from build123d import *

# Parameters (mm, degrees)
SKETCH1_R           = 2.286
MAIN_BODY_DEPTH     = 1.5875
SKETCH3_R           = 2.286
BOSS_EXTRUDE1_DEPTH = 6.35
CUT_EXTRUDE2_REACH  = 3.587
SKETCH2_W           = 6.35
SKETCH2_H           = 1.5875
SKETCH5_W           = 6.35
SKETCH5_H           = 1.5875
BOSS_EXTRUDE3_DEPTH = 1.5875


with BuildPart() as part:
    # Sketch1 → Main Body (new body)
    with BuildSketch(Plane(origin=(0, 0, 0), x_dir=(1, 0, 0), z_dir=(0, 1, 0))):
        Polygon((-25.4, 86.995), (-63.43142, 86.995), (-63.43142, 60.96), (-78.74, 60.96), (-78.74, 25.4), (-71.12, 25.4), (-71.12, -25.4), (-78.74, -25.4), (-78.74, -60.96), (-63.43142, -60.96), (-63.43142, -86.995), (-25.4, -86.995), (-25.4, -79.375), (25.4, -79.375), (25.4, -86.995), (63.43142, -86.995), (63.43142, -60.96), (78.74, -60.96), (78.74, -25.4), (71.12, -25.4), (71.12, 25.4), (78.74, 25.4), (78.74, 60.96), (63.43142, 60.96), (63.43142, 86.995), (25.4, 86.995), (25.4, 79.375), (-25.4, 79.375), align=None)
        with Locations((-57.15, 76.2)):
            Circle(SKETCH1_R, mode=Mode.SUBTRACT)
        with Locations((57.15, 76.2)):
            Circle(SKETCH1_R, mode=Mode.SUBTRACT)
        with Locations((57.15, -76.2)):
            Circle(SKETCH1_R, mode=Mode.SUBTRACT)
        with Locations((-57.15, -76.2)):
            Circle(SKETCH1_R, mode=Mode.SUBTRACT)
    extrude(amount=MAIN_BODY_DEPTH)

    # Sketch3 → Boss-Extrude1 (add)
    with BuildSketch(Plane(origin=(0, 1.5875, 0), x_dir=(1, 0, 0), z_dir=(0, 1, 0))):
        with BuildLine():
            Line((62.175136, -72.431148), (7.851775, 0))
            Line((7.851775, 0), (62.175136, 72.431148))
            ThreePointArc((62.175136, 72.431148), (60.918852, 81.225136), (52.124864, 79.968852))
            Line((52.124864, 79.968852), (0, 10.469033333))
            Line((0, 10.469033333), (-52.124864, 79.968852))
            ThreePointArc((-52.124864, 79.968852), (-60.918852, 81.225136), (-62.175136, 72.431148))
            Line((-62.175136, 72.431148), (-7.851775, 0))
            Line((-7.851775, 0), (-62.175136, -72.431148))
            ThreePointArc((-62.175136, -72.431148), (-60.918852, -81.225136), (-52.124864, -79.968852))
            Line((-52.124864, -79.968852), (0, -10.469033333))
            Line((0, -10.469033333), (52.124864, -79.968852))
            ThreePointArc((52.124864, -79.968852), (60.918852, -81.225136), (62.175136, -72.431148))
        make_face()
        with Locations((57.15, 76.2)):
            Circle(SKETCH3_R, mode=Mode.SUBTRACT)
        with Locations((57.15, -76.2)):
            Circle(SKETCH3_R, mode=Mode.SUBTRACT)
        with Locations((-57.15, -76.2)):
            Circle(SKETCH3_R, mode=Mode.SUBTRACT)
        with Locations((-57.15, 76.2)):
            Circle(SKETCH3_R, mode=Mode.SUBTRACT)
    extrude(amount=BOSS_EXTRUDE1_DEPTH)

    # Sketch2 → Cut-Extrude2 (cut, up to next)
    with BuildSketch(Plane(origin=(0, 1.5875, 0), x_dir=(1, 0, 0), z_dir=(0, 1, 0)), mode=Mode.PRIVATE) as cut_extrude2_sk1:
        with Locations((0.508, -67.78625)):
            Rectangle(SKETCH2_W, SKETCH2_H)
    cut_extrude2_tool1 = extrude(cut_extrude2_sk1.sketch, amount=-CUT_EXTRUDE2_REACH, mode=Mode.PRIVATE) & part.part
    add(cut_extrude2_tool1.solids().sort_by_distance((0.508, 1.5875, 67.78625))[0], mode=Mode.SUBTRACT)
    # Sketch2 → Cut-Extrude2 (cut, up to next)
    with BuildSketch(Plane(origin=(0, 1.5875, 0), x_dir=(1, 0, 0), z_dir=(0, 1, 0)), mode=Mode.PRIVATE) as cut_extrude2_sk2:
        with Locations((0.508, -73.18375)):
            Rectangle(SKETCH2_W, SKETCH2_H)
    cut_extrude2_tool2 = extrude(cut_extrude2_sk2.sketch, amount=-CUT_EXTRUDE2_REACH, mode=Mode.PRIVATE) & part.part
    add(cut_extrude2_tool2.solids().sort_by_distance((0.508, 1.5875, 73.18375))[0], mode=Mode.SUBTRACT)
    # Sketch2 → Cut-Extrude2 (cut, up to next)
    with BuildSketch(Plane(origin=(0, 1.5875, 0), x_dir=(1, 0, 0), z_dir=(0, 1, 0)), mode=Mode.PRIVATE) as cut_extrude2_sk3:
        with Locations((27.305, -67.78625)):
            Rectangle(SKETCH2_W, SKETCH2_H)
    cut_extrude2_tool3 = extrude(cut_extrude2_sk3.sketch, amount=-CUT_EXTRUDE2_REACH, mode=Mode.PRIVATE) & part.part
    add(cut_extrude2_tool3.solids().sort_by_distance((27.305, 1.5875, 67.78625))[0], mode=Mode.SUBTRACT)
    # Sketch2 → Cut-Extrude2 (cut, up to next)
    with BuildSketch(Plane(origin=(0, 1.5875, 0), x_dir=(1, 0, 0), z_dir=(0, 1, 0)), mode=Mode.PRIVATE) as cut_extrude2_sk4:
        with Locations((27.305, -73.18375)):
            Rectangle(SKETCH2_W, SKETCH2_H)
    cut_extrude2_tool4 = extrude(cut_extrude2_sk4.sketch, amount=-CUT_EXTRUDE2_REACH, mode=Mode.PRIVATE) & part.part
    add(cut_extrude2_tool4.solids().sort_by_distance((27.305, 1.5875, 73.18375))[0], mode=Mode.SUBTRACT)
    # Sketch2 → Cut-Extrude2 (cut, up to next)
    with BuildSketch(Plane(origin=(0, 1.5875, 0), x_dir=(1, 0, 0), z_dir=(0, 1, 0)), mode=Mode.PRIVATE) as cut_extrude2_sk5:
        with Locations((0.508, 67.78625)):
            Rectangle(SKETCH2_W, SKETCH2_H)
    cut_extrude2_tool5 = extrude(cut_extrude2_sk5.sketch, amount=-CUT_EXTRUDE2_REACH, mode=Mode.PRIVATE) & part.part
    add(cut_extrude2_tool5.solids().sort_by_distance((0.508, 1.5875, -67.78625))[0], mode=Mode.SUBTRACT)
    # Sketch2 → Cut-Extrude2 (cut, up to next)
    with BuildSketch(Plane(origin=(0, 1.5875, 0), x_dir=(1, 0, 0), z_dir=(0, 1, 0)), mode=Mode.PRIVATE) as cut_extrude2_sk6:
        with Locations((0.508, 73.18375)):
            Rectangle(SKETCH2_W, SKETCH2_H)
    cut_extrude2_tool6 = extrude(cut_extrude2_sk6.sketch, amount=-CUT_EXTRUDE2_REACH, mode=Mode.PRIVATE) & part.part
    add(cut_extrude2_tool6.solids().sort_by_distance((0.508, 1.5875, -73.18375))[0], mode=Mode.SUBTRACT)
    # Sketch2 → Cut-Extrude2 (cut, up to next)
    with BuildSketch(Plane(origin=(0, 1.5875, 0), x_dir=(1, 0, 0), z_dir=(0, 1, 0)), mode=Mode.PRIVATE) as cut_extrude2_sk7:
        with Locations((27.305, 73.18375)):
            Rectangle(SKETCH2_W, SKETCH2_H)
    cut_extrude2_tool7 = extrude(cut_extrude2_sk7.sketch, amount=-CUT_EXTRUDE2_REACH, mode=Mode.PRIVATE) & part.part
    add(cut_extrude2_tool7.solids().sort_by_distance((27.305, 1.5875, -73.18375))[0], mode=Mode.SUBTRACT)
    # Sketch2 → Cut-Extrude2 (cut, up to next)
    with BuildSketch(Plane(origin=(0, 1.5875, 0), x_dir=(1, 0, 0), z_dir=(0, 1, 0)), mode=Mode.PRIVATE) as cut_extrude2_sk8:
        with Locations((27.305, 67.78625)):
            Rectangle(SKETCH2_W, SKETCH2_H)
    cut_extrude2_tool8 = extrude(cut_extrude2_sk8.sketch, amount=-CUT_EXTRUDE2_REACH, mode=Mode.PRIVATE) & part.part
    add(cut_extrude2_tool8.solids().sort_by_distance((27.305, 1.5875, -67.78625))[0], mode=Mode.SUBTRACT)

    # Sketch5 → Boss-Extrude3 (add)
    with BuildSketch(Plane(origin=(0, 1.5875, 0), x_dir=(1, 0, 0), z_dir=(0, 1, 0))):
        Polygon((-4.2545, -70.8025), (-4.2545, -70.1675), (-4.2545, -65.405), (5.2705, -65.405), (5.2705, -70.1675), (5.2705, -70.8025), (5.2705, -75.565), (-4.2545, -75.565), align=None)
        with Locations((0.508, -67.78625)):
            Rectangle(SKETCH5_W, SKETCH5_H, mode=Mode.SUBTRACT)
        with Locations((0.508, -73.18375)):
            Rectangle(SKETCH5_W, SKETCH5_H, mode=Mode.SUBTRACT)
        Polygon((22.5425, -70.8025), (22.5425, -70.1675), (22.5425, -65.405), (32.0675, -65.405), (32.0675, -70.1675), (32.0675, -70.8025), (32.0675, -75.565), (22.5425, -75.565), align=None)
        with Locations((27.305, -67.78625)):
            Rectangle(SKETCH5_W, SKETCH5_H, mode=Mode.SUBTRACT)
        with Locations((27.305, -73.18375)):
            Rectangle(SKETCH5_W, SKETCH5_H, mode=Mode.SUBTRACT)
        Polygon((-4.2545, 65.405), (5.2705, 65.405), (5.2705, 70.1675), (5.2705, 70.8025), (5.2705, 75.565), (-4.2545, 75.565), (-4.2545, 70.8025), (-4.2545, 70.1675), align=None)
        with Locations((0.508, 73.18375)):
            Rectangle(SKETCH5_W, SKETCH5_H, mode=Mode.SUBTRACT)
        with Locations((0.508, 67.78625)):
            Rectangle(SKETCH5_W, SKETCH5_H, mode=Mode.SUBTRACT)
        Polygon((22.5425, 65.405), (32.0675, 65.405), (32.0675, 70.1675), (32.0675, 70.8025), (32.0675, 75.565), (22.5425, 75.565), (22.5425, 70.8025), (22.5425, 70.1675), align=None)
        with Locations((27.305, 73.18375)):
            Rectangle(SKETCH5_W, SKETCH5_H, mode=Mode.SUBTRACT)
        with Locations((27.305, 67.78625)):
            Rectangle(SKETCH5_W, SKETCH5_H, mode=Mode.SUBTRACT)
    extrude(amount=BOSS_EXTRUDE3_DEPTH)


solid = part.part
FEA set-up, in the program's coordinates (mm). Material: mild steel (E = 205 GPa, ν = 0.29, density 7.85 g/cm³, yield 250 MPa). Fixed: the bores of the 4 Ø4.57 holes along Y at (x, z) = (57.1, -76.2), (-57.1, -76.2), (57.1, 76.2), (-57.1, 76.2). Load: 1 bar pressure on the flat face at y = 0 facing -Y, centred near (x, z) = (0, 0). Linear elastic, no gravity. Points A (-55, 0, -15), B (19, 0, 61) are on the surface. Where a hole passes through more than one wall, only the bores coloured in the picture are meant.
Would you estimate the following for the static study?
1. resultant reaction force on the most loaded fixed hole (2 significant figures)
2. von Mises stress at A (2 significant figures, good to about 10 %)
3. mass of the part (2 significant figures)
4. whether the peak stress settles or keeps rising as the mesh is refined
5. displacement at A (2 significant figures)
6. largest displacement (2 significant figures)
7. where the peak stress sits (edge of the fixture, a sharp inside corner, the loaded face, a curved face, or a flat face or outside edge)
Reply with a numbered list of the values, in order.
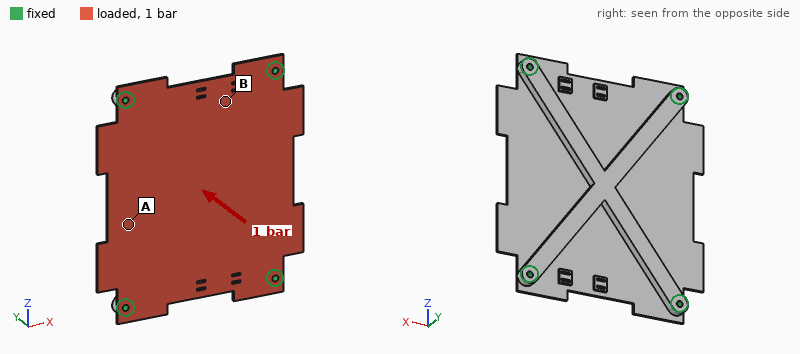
1. 990 N
2. 54 MPa
3. 540 g
4. keeps rising
5. 0.29 mm
6. 0.50 mm
7. edge of the fixture
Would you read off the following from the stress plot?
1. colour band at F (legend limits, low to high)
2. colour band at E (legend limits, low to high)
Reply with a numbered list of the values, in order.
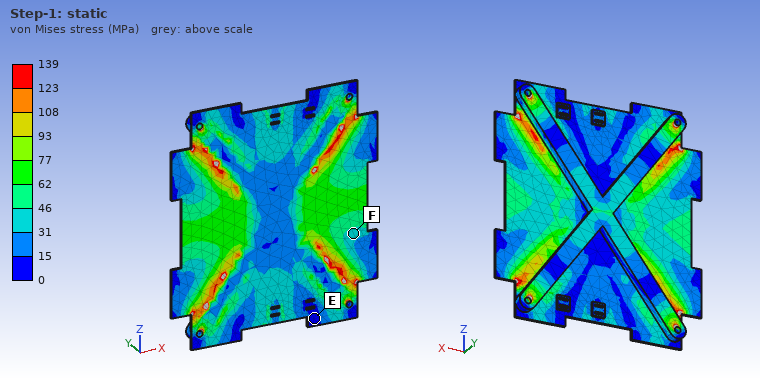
1. 31 to 46 MPa
2. 0 to 15 MPa
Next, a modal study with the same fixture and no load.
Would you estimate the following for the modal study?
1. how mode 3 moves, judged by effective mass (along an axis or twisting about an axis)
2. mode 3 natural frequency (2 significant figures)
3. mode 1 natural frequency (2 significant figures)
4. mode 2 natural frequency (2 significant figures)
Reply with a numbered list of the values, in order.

1. along Y
2. 1300 Hz
3. 870 Hz
4. 880 Hz
